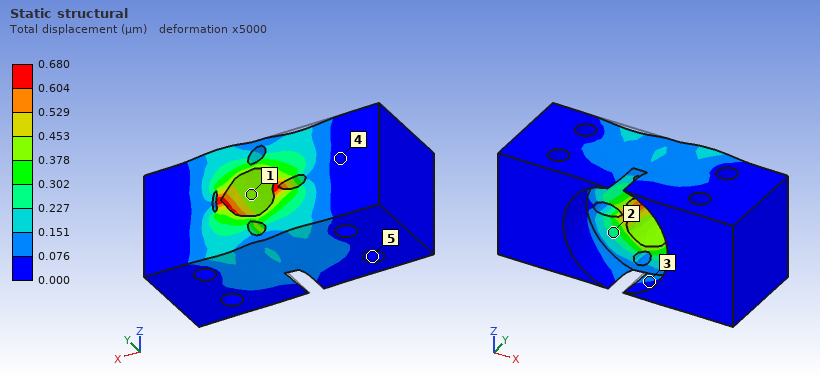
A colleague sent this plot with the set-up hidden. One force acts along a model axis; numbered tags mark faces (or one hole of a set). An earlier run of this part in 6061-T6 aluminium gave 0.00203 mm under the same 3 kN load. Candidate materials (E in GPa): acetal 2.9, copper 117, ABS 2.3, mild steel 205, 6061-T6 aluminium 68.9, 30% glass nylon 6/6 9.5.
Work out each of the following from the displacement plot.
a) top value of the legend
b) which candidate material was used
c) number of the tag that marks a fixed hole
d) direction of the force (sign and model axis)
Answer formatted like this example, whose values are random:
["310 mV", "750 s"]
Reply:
["0.680 µm", "mild steel", "5", "+X"]
